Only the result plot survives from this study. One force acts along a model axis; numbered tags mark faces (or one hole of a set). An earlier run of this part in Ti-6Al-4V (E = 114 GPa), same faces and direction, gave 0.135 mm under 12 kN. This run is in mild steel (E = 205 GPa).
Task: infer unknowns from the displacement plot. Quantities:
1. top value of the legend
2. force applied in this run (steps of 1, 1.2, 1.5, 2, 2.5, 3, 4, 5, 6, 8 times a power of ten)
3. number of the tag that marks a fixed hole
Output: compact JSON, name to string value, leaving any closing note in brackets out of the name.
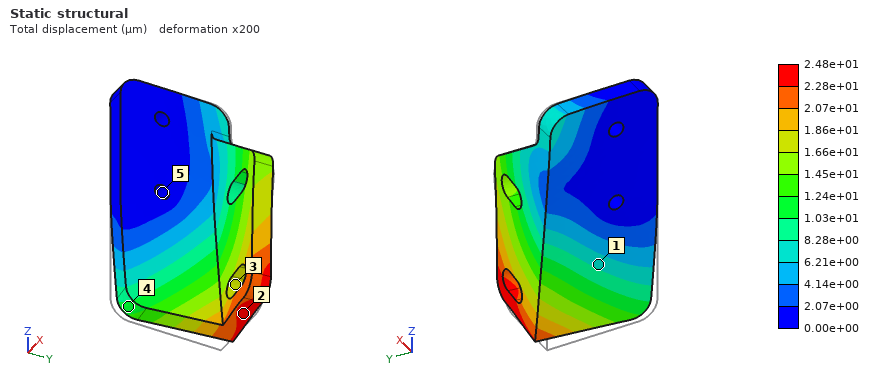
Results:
{"top value of the legend": "2.48e+01 µm", "force applied in this run": "4 kN", "number of the tag that marks a fixed hole": "5"}
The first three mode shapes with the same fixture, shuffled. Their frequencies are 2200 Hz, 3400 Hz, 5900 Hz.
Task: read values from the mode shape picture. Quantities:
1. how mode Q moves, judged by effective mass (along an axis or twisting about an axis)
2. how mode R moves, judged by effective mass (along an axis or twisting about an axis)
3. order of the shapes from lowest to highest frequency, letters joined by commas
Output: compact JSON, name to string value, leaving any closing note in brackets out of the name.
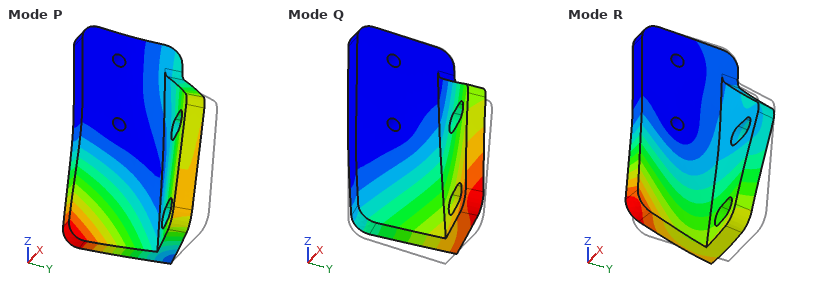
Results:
{"how mode Q moves, judged by effective mass": "along X", "how mode R moves, judged by effective mass": "along Y", "order of the shapes from lowest to highest frequency, letters joined by commas": "Q, P, R"}
